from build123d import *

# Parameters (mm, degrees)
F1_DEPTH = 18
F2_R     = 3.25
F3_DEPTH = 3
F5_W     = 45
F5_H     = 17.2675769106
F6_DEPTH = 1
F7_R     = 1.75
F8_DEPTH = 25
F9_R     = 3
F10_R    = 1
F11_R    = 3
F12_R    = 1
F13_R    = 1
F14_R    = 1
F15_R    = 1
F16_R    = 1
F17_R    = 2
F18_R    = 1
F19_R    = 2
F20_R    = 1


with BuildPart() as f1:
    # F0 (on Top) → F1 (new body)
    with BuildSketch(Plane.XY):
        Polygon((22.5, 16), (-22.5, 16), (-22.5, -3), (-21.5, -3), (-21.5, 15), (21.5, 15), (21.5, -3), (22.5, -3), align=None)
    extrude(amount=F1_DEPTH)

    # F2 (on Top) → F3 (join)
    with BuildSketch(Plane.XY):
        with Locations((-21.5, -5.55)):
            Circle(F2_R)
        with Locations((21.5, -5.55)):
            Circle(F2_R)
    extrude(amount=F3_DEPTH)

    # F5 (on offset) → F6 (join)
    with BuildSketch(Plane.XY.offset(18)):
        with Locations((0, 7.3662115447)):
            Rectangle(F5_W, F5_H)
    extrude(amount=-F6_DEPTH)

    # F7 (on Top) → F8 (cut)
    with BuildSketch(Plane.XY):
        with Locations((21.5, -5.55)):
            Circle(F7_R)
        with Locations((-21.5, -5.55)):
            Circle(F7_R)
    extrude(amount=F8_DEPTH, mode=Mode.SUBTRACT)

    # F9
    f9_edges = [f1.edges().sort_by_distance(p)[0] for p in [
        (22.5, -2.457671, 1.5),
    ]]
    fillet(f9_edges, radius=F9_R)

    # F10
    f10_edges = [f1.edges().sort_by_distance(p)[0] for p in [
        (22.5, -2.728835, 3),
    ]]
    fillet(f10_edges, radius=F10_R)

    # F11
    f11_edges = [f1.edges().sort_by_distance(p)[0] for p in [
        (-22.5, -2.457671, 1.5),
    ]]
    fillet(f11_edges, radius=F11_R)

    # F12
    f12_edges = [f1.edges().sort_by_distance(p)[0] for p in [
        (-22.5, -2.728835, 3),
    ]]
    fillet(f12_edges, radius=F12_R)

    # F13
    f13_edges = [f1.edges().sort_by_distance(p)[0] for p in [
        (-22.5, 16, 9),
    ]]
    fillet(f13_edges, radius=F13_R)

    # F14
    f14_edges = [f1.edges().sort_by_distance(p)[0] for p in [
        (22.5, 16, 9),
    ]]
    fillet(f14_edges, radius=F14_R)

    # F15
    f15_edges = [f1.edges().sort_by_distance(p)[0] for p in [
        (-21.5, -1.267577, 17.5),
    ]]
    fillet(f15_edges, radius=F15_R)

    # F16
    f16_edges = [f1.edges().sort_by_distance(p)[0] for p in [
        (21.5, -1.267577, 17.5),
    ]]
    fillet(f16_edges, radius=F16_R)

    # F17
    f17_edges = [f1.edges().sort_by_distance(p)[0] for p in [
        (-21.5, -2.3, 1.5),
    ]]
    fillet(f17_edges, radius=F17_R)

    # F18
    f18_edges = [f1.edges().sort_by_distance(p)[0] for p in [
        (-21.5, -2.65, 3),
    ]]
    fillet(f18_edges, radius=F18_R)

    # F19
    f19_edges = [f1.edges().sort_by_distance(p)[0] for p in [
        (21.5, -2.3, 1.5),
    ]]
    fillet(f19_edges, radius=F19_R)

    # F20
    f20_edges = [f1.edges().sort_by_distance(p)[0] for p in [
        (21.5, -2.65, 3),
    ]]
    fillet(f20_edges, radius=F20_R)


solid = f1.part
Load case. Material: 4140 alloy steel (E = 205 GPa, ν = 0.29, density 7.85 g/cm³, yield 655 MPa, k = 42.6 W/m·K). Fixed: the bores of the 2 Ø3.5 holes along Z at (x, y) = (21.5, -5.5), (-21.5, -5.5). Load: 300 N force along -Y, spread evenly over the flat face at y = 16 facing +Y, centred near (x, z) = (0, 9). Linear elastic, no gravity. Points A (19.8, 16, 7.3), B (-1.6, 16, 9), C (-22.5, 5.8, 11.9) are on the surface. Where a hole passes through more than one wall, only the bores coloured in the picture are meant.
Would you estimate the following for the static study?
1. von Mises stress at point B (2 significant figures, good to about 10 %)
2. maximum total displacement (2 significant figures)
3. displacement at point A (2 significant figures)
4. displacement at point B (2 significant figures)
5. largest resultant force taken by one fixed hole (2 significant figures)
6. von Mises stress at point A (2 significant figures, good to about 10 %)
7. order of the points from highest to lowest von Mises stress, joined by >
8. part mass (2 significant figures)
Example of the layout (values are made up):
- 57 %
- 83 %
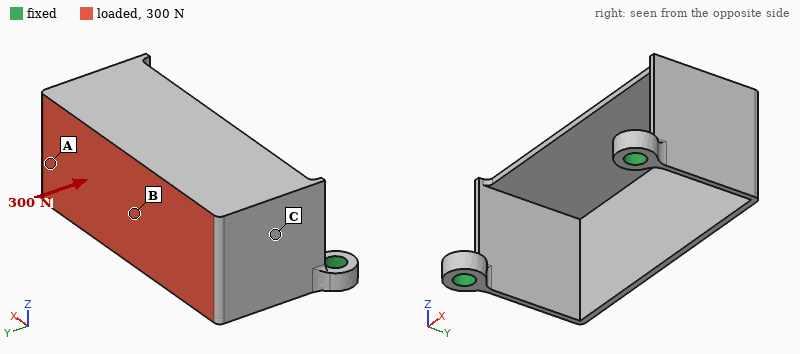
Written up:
- 56 MPa
- 0.19 mm
- 0.075 mm
- 0.13 mm
- 150 N
- 110 MPa
- A > B > C
- 18 g
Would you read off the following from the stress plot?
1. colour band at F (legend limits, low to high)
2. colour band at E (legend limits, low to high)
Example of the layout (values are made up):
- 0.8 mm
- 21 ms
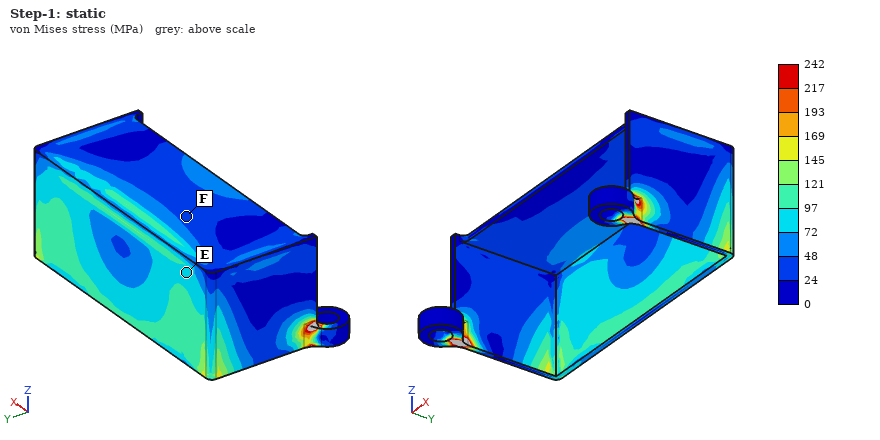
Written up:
- 24 to 48 MPa
- 72 to 97 MPa
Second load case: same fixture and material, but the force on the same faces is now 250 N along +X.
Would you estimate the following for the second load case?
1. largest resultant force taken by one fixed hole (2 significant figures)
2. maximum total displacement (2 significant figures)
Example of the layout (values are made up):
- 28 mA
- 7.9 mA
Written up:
- 150 N
- 0.29 mm
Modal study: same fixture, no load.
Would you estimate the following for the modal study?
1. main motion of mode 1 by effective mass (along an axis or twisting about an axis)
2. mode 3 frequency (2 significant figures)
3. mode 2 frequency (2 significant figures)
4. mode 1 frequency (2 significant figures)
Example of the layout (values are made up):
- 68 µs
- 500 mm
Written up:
- along X
- 2500 Hz
- 1600 Hz
- 1300 Hz
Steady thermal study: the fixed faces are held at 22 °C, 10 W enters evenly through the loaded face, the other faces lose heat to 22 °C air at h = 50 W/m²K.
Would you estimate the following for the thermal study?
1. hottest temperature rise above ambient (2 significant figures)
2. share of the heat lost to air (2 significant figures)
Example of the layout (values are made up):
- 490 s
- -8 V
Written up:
- 77 K
- 80 %
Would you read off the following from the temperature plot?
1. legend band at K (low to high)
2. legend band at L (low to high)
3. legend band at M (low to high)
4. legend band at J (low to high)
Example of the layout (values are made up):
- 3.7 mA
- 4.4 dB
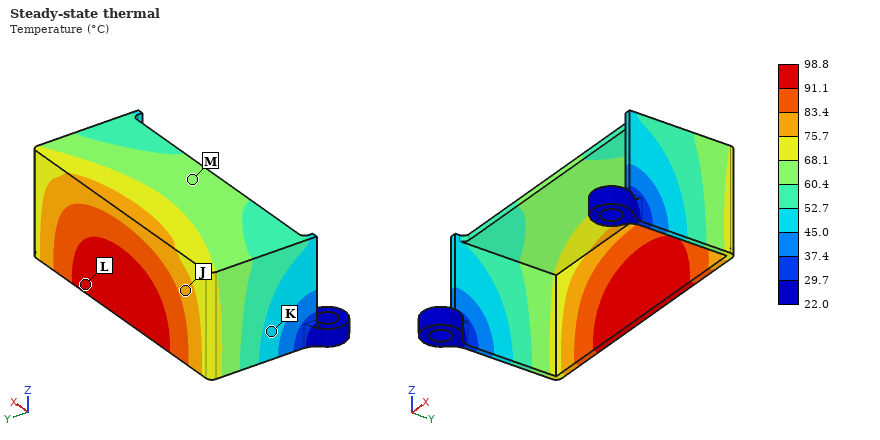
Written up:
- 45.0 to 52.7 °C
- 91.1 to 98.8 °C
- 60.4 to 68.1 °C
- 75.7 to 83.4 °C
